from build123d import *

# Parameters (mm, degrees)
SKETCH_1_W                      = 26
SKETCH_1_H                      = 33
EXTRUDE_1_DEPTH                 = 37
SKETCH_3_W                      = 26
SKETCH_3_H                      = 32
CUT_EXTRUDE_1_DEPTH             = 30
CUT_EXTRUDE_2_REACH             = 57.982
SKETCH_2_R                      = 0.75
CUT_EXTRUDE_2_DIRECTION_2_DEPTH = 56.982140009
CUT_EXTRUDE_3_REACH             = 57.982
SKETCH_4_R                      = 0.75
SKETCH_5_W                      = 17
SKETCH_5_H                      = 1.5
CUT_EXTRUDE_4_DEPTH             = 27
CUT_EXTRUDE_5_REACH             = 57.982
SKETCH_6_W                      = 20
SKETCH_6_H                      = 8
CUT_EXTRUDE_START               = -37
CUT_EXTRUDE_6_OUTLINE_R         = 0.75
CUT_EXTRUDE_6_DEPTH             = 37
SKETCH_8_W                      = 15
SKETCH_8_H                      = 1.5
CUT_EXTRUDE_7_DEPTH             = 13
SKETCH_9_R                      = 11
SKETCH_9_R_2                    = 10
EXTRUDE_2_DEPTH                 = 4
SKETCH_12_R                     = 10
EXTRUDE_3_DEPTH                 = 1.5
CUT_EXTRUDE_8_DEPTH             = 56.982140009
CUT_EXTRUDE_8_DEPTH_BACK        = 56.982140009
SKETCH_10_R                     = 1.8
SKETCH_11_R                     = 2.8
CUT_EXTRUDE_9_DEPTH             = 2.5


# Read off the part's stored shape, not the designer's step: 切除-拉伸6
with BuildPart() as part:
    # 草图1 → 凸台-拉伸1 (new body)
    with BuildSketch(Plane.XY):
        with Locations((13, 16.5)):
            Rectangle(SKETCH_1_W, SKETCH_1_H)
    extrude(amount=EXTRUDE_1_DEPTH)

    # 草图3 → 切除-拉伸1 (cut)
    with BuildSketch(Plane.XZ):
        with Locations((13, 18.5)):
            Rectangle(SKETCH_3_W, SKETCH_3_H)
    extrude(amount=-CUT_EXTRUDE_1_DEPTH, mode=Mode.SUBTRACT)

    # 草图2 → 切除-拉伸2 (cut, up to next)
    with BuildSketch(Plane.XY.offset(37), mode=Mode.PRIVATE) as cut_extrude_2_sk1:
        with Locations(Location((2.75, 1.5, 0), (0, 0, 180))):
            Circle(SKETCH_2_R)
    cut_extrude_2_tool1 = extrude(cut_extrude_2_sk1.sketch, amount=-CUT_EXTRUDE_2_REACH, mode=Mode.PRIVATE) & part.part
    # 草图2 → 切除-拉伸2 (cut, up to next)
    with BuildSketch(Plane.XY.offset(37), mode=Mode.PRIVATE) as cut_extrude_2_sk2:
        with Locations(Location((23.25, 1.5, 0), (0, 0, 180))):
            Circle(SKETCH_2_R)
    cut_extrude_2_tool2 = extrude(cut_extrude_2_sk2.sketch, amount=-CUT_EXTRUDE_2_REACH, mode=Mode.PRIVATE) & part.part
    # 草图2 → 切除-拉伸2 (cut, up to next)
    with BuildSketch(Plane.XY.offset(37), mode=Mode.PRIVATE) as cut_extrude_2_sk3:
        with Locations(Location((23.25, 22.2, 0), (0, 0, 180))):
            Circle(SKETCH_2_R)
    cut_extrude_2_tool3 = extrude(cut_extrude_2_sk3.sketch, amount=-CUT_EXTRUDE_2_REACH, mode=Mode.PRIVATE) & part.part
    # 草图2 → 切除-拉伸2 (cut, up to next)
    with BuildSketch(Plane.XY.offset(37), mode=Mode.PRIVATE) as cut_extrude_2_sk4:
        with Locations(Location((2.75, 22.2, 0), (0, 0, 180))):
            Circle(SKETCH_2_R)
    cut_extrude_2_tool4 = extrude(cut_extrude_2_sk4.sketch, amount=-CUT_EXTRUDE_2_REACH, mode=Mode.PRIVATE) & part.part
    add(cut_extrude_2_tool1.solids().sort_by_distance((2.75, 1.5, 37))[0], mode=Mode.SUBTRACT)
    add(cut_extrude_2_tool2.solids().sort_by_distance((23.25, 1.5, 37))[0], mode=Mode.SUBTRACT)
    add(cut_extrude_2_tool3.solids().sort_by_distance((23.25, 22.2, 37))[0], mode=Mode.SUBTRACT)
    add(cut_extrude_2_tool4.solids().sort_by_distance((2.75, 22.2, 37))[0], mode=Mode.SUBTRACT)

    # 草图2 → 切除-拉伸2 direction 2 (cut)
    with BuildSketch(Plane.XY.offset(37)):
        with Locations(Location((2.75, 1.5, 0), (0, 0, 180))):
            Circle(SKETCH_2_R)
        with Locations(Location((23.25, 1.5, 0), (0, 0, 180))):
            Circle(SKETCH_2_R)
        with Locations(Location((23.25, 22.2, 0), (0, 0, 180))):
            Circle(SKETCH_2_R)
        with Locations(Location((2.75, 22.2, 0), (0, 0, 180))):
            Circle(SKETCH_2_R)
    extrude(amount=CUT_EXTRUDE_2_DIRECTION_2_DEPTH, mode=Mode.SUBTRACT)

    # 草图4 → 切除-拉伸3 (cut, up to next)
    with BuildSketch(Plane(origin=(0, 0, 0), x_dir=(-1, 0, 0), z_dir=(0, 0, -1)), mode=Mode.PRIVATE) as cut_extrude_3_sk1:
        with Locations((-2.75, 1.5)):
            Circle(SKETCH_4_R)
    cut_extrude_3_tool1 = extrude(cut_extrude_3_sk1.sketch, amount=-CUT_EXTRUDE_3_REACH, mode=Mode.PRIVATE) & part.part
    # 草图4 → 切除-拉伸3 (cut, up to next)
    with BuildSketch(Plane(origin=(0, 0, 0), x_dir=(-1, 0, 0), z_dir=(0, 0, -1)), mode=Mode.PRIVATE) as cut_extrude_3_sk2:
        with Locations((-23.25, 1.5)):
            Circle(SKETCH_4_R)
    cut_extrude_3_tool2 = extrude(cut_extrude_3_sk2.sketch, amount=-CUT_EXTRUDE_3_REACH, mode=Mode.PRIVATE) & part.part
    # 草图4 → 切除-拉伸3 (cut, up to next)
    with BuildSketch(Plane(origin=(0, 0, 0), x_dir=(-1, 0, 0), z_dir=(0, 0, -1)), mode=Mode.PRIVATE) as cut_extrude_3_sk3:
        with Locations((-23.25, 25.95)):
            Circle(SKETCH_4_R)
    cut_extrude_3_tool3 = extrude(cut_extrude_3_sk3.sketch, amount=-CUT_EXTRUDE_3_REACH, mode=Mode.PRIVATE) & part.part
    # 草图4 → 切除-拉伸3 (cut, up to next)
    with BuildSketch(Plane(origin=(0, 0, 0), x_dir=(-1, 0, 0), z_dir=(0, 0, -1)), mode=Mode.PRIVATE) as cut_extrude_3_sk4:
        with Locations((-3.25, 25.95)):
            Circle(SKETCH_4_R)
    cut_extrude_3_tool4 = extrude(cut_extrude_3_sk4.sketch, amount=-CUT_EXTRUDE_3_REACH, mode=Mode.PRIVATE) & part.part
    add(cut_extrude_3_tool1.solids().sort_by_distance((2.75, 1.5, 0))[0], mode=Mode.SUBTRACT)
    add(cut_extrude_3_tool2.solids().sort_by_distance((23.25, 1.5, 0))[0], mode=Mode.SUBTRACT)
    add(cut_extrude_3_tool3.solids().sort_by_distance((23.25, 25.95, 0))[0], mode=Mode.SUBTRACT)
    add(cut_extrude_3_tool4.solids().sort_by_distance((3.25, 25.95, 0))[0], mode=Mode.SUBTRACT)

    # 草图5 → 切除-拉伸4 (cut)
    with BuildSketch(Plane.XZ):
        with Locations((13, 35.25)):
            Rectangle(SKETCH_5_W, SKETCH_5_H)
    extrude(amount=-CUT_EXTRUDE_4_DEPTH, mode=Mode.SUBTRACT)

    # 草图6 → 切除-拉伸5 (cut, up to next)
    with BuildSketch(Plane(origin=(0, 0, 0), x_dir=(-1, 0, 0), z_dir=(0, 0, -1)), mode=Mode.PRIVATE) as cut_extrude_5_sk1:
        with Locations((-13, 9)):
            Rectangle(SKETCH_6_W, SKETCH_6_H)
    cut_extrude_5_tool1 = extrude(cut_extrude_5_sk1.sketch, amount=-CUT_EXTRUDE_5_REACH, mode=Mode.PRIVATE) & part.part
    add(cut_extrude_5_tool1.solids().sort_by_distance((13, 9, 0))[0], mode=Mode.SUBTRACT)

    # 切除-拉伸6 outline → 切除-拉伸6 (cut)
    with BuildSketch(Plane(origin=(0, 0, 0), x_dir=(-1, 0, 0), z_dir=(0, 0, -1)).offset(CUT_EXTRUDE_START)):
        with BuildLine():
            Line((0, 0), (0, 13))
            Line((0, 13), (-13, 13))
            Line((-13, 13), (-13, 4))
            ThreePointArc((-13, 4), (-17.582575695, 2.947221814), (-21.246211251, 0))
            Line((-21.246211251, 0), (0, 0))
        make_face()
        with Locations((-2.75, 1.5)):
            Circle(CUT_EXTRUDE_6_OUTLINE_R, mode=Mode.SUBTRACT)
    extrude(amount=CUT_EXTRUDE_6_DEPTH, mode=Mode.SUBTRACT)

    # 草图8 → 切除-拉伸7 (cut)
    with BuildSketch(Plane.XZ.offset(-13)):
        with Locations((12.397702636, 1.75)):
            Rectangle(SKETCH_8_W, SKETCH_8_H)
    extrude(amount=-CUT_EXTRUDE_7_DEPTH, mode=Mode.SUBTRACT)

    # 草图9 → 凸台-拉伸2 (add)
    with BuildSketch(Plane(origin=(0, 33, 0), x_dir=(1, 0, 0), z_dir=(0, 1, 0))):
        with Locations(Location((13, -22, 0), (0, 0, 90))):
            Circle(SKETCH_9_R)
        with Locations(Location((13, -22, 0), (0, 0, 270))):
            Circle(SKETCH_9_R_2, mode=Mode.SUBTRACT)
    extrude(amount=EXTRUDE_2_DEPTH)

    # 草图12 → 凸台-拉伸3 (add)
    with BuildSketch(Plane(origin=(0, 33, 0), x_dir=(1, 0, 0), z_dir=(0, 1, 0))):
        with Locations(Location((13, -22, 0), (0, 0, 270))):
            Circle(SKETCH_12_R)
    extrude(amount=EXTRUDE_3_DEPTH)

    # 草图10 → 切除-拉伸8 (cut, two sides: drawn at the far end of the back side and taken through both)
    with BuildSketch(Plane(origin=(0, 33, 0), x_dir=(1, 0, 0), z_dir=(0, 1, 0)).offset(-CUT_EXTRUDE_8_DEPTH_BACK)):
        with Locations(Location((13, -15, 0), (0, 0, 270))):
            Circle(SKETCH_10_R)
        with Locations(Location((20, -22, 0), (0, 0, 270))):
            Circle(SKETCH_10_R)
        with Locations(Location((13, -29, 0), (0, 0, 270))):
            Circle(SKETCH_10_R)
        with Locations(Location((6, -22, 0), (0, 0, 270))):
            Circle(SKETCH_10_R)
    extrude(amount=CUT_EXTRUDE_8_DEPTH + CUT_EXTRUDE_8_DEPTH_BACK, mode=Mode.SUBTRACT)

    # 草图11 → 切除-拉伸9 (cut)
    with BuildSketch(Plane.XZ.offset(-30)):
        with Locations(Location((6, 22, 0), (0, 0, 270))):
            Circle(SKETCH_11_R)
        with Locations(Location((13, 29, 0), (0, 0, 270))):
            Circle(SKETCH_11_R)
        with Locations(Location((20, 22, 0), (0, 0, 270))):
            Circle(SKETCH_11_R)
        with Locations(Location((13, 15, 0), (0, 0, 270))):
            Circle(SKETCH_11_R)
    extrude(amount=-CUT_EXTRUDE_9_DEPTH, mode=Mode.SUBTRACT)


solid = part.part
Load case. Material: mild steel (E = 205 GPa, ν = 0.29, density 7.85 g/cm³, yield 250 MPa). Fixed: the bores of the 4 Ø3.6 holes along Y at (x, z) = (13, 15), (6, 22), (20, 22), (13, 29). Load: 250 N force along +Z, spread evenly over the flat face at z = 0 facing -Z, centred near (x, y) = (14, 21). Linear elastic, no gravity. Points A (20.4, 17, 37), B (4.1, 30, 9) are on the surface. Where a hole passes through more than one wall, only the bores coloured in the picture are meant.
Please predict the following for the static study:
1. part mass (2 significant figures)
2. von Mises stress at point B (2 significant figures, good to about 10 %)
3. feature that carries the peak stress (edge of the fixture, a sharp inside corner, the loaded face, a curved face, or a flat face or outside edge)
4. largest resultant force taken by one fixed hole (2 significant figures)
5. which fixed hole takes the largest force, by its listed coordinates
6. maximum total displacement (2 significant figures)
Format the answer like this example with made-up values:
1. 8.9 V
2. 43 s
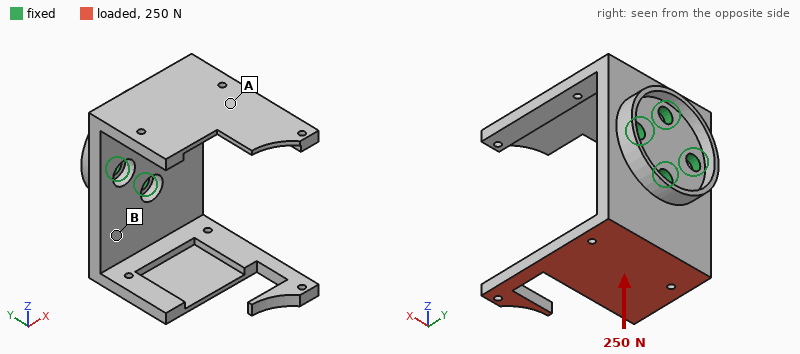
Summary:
1. 41 g
2. 64 MPa
3. a curved face
4. 360 N
5. (13, 15)
6. 0.25 mm
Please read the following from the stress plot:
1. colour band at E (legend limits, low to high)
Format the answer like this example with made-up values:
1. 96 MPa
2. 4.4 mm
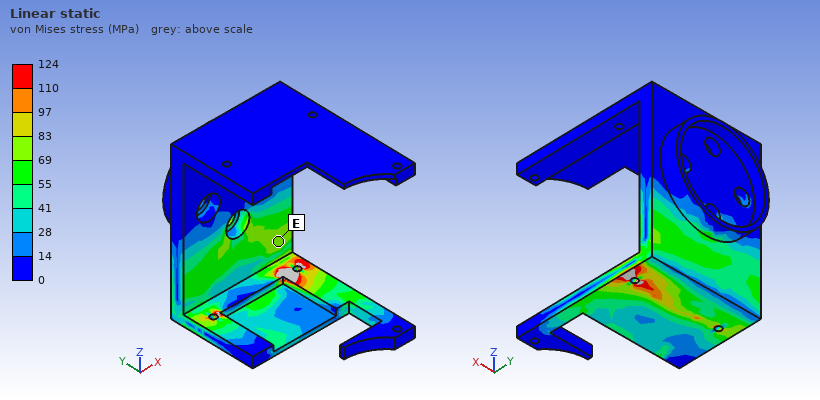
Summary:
1. 69 to 83 MPa
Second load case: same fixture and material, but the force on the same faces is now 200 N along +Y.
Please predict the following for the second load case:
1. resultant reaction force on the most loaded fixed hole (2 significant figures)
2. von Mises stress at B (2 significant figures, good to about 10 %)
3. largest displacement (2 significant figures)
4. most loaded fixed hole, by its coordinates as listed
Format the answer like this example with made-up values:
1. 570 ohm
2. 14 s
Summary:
1. 510 N
2. 42 MPa
3. 76 µm
4. (13, 15)
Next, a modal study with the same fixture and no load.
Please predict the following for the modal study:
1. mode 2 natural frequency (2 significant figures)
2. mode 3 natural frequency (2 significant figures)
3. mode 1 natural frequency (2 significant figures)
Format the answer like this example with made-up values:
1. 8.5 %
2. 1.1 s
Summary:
1. 2200 Hz
2. 3900 Hz
3. 2100 Hz
